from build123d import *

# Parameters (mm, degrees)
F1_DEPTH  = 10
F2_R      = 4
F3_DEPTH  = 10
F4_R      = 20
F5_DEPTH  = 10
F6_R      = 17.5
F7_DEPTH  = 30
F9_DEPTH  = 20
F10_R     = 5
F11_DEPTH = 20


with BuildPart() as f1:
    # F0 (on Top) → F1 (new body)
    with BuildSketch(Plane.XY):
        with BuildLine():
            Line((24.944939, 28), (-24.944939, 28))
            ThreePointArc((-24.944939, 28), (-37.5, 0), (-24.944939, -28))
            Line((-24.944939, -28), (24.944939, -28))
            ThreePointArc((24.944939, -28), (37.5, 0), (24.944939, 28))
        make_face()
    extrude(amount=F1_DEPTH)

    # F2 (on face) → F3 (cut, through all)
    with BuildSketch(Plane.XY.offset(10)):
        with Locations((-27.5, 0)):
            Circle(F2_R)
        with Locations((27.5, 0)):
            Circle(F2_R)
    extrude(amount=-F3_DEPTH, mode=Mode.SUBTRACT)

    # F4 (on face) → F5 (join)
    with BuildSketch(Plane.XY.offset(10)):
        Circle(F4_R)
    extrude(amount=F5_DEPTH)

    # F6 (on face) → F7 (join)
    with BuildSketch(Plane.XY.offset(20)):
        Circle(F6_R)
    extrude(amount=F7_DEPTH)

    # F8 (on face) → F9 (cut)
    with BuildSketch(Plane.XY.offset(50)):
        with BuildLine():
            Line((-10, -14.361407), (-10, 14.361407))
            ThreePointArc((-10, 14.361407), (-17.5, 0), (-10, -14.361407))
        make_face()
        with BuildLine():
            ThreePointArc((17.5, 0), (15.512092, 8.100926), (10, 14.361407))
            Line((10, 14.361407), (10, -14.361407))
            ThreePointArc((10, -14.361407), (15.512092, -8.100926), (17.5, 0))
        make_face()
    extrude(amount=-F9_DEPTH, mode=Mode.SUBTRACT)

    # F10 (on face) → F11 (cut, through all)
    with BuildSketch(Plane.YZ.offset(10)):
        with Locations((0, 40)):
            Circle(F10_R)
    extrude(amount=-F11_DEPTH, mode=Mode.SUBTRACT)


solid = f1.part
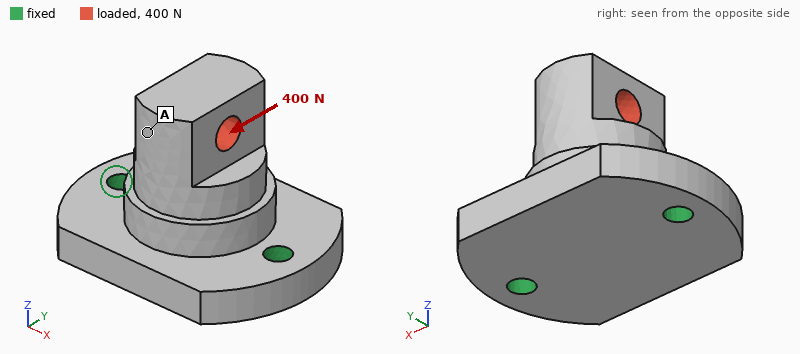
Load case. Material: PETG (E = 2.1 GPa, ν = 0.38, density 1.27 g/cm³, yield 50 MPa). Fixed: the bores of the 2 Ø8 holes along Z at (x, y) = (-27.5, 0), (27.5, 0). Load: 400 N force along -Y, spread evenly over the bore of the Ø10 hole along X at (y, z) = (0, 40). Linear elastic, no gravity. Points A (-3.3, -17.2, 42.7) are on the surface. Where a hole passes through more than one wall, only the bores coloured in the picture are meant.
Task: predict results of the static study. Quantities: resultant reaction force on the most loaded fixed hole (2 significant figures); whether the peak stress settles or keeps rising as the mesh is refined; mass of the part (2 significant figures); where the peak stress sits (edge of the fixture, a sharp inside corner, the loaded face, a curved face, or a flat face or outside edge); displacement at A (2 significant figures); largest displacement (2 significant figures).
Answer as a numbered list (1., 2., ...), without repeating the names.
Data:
1. 200 N
2. keeps rising
3. 90 g
4. edge of the fixture
5. 0.42 mm
6. 0.49 mm
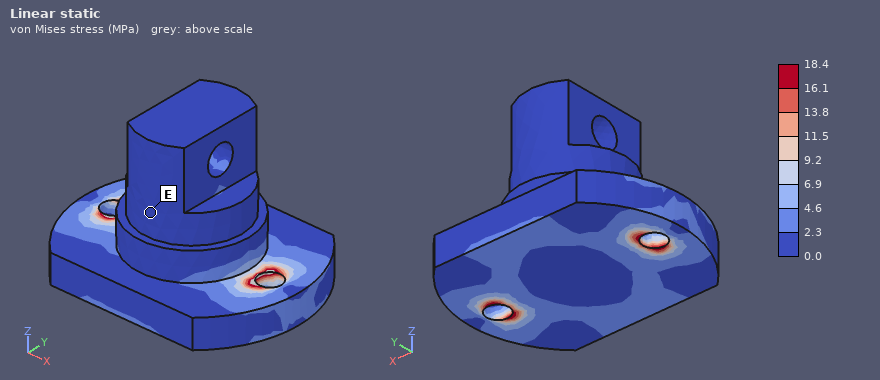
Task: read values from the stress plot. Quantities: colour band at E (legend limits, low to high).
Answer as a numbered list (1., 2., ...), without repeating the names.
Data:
1. 0.0 to 2.3 MPa
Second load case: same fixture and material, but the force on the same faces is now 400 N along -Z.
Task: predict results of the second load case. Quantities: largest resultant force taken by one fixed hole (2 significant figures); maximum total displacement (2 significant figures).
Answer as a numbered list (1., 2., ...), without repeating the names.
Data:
1. 220 N
2. 36 µm
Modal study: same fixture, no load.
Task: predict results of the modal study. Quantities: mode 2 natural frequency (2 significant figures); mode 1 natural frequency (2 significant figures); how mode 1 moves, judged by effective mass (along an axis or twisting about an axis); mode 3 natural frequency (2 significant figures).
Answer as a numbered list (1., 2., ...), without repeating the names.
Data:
1. 2500 Hz
2. 1000 Hz
3. along Y
4. 2500 Hz
